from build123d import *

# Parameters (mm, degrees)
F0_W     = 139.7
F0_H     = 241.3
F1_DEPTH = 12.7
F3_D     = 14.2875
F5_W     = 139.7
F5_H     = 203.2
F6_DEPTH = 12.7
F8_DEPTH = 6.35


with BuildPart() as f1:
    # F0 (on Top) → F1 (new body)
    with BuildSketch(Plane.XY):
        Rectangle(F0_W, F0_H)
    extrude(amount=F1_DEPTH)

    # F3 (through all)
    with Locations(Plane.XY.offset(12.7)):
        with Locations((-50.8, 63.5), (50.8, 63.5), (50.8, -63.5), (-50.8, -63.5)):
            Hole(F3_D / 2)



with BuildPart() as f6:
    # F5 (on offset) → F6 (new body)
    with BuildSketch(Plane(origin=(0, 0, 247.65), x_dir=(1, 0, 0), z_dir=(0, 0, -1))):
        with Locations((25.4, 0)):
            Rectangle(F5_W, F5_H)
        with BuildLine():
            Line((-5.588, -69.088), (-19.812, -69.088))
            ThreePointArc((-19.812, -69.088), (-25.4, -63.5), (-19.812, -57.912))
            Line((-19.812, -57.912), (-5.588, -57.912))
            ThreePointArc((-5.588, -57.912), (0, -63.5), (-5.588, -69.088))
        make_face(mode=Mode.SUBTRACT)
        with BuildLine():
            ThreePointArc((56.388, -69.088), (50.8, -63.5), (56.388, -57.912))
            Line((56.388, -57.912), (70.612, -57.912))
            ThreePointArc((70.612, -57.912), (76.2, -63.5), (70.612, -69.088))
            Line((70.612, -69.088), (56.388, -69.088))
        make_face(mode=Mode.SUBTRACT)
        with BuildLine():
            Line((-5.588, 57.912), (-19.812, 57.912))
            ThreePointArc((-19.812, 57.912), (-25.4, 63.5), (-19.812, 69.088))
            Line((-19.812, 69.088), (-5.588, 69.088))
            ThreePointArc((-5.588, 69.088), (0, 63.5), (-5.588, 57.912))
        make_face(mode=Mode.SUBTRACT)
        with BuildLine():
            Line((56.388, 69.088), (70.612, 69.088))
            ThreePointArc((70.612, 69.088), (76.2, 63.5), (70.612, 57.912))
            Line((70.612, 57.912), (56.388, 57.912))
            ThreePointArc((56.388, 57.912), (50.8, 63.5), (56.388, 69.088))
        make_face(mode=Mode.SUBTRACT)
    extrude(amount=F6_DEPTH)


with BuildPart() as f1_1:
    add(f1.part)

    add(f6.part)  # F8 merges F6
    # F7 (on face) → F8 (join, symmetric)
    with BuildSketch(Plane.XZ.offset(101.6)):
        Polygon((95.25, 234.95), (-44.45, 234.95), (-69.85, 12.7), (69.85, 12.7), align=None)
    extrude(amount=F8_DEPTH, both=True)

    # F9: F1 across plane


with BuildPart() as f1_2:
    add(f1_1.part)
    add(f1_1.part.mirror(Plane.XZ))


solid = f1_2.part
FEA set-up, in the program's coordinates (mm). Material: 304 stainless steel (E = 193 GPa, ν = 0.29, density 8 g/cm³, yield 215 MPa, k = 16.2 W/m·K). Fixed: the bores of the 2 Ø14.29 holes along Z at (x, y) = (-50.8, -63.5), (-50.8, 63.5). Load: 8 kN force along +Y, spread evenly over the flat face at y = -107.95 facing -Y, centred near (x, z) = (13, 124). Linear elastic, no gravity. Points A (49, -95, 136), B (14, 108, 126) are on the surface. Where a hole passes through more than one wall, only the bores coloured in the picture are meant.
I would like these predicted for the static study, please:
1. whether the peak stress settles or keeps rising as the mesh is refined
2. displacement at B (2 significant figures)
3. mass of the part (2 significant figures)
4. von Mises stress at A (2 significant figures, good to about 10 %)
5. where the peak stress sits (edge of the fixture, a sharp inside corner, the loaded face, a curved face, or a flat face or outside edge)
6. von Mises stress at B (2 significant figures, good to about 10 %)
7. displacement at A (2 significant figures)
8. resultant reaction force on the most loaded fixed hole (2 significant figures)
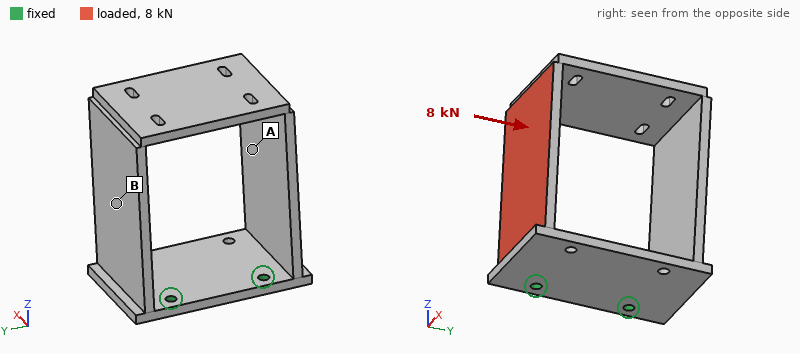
keeps rising
0.58 mm
12 kg
38 MPa
edge of the fixture
12 MPa
0.78 mm
7.0 kN
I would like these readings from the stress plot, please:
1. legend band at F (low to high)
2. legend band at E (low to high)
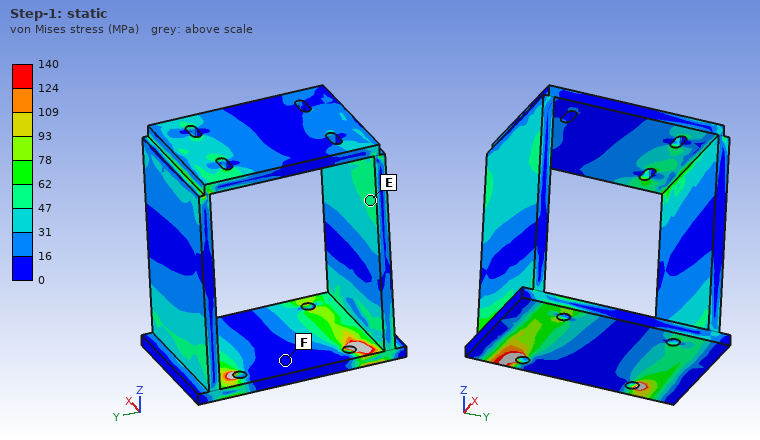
0 to 16 MPa
47 to 62 MPa
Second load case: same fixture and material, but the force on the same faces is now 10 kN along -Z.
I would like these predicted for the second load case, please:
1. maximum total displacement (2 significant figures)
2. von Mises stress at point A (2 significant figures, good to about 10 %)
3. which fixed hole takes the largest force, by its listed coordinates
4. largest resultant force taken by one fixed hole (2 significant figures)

0.90 mm
16 MPa
(-50.8, -63.5)
11 kN
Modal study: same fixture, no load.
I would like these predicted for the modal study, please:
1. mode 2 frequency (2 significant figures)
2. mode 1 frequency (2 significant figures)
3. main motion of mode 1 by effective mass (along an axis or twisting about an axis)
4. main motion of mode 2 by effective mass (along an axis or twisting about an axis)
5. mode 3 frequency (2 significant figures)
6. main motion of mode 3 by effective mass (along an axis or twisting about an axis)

140 Hz
130 Hz
along Y
along X
320 Hz
twisting about Z
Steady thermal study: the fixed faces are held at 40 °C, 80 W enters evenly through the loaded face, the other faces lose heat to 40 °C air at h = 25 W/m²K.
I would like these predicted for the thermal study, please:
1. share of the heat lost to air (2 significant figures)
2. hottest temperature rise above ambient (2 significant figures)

91 %
62 K
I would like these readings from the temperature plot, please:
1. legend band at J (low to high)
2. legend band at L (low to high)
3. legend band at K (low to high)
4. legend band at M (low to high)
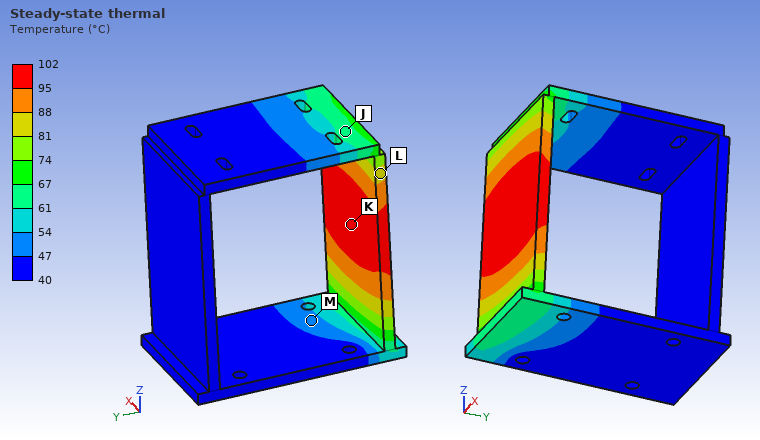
61 to 67 °C
81 to 88 °C
95 to 102 °C
47 to 54 °C
